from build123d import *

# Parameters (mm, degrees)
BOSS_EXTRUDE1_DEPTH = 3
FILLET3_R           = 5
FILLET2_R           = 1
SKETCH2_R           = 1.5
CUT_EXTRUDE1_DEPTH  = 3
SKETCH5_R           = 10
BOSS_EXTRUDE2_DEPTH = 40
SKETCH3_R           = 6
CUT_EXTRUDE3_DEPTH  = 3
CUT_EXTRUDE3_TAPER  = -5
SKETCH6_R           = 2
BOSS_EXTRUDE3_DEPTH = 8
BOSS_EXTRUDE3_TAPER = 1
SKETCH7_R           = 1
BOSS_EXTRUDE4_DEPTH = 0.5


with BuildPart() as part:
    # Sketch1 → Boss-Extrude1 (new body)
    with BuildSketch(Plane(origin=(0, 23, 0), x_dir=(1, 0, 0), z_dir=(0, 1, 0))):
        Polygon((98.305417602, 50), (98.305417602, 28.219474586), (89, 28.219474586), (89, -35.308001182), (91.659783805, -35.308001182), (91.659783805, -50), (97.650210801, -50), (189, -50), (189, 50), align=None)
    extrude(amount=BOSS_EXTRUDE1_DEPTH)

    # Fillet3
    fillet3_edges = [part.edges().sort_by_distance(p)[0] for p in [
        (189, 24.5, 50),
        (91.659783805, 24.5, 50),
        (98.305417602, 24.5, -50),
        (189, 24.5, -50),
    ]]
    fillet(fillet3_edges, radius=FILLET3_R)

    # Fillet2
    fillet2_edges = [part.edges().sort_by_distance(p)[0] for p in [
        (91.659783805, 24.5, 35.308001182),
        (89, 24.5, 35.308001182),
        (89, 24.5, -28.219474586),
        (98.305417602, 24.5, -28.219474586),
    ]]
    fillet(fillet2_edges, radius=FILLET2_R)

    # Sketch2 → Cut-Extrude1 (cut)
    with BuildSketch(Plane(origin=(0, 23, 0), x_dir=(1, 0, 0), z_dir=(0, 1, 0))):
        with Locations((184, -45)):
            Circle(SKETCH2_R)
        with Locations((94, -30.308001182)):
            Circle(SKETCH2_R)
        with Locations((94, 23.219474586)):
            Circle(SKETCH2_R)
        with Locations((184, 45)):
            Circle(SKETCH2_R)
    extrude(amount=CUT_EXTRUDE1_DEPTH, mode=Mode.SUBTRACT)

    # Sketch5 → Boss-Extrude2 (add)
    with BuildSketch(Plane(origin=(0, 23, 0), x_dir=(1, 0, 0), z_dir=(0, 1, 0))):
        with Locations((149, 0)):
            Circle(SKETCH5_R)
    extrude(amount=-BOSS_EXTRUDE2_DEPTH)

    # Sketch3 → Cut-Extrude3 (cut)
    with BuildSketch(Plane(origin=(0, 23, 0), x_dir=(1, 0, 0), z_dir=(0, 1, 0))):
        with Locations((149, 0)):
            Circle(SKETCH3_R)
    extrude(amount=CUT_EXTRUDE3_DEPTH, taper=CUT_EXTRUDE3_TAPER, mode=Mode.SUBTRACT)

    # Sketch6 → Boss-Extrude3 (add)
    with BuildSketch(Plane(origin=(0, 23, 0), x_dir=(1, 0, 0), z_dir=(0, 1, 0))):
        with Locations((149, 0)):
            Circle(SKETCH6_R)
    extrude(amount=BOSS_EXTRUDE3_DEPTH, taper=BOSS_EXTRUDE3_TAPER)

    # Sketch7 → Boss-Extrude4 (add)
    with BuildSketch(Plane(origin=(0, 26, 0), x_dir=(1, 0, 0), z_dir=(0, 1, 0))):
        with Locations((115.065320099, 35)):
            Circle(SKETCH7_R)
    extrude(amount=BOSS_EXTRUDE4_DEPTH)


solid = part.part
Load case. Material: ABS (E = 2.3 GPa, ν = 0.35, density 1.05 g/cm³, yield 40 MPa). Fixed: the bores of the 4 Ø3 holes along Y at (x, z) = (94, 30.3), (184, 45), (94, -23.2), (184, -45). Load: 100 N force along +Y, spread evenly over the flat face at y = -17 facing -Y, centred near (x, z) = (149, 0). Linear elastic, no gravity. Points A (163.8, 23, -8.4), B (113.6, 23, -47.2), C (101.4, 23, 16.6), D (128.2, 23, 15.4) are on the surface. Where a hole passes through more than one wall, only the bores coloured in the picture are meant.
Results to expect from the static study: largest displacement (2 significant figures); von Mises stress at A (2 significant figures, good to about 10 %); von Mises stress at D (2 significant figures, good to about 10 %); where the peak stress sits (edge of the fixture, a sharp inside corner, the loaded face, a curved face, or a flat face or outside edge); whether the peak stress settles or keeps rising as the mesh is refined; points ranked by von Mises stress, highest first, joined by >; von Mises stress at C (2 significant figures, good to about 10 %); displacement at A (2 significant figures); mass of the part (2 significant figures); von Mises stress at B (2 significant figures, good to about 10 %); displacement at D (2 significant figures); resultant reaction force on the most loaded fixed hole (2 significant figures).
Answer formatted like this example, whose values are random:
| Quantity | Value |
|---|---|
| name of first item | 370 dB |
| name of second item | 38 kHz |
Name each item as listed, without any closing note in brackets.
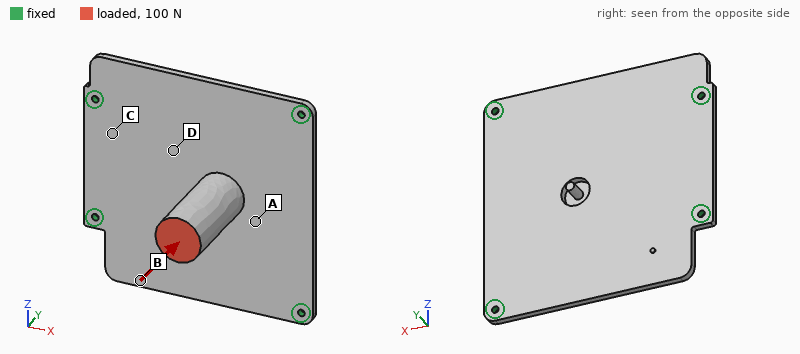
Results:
| Quantity | Value |
|---|---|
| largest displacement | 1.5 mm |
| von Mises stress at A | 7.5 MPa |
| von Mises stress at D | 4.6 MPa |
| where the peak stress sits | edge of the fixture |
| whether the peak stress settles or keeps rising as the mesh is refined | keeps rising |
| points ranked by von Mises stress, highest first, joined by > | A > D > C > B |
| von Mises stress at C | 3.4 MPa |
| displacement at A | 1.4 mm |
| mass of the part | 44 g |
| von Mises stress at B | 1.3 MPa |
| displacement at D | 1.1 mm |
| resultant reaction force on the most loaded fixed hole | 31 N |
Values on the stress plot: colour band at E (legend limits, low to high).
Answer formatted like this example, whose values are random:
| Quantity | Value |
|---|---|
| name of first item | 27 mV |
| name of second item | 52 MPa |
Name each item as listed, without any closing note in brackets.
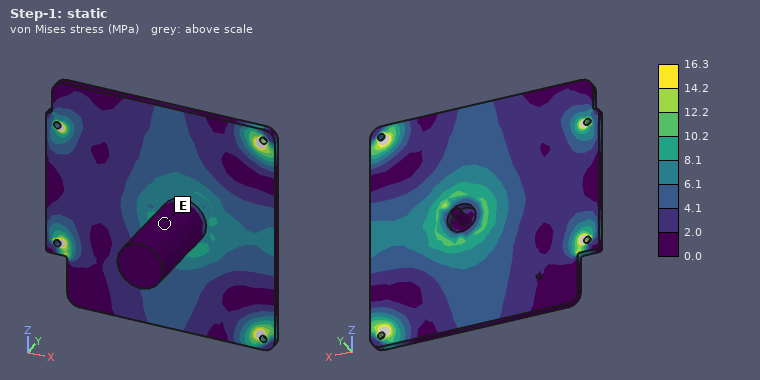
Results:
| Quantity | Value |
|---|---|
| colour band at E | 0.0 to 2.0 MPa |
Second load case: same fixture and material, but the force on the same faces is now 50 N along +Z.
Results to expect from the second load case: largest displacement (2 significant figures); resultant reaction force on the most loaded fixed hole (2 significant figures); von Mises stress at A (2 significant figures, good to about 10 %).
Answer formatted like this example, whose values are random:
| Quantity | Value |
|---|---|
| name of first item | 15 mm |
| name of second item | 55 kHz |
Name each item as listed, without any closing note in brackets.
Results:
| Quantity | Value |
|---|---|
| largest displacement | 1.7 mm |
| resultant reaction force on the most loaded fixed hole | 25 N |
| von Mises stress at A | 6.4 MPa |
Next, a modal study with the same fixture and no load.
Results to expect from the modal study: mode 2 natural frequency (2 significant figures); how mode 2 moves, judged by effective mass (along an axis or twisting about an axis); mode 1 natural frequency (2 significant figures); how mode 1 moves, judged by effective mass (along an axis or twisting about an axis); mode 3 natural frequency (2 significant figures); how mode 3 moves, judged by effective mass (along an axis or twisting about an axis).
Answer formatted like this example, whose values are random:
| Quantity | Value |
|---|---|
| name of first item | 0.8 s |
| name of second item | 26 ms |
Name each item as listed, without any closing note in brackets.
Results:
| Quantity | Value |
|---|---|
| mode 2 natural frequency | 360 Hz |
| how mode 2 moves, judged by effective mass | along Z |
| mode 1 natural frequency | 270 Hz |
| how mode 1 moves, judged by effective mass | along Y |
| mode 3 natural frequency | 370 Hz |
| how mode 3 moves, judged by effective mass | along X |
